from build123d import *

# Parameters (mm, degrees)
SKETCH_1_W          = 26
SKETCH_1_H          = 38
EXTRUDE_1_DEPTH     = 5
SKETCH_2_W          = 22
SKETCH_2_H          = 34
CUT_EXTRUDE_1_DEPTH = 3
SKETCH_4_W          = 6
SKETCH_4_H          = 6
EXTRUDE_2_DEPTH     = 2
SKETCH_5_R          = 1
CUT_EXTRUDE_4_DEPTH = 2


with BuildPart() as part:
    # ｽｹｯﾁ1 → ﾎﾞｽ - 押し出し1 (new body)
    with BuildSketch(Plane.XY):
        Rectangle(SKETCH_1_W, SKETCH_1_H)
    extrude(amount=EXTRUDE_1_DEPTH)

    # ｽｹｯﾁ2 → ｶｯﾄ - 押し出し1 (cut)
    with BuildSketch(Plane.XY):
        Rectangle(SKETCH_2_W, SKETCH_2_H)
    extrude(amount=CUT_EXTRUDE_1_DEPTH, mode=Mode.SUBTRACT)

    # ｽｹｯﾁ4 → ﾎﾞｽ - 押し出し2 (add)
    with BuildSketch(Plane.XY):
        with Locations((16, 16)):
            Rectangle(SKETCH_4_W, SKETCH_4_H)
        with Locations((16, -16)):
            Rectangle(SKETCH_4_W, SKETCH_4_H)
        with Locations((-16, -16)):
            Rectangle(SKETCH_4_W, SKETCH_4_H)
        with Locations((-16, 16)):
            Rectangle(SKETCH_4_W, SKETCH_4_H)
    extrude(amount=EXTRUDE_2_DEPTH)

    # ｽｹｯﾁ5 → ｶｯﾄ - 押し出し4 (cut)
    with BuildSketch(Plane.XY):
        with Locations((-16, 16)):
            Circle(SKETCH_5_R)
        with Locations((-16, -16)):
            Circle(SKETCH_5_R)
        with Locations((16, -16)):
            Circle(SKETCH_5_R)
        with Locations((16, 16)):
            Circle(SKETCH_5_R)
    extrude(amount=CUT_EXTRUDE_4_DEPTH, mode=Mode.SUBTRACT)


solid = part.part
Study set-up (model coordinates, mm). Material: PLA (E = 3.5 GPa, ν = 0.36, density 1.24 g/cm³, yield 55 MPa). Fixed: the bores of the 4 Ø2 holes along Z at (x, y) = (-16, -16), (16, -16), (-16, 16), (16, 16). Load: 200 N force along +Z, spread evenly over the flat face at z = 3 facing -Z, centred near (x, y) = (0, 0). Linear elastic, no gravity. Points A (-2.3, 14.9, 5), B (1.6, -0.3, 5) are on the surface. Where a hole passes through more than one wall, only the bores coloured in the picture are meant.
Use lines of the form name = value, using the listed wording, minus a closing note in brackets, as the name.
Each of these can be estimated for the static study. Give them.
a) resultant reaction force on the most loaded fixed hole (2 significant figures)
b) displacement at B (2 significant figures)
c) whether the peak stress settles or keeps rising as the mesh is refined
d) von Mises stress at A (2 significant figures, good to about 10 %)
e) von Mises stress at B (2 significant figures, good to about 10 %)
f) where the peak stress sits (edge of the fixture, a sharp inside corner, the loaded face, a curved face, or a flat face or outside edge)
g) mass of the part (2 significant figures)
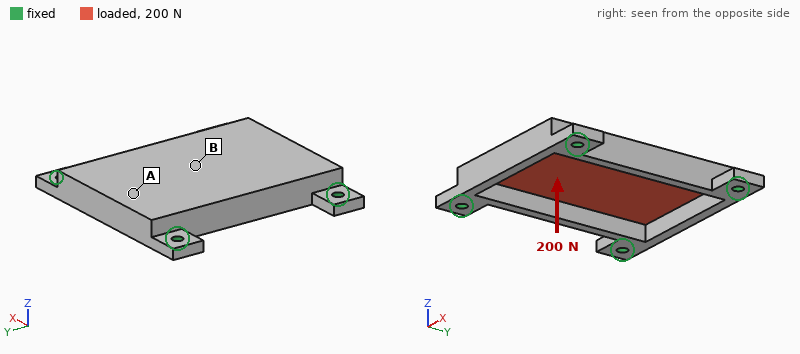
resultant reaction force on the most loaded fixed hole = 96 N
displacement at B = 0.30 mm
whether the peak stress settles or keeps rising as the mesh is refined = keeps rising
von Mises stress at A = 8.1 MPa
von Mises stress at B = 15 MPa
where the peak stress sits = edge of the fixture
mass of the part = 3.7 g
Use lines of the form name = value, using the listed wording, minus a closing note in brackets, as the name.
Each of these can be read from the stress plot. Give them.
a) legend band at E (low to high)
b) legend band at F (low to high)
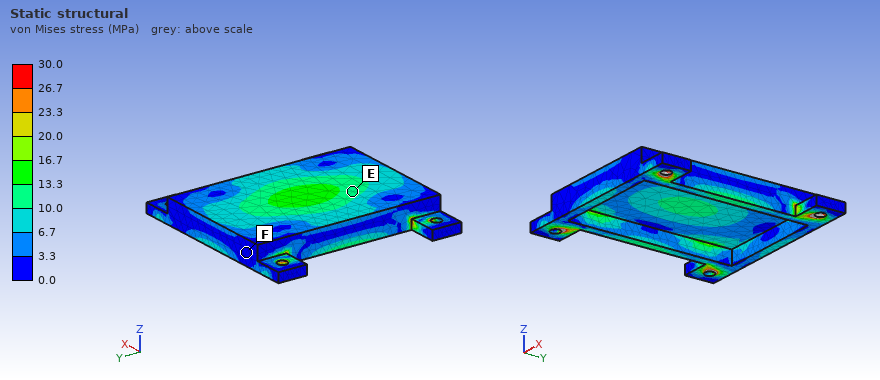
legend band at E = 10.0 to 13.3 MPa
legend band at F = 0.0 to 3.3 MPa
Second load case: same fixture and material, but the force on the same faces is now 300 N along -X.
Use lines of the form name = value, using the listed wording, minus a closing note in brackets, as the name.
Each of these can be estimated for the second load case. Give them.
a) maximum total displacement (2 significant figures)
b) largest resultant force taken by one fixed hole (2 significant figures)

maximum total displacement = 84 µm
largest resultant force taken by one fixed hole = 76 N
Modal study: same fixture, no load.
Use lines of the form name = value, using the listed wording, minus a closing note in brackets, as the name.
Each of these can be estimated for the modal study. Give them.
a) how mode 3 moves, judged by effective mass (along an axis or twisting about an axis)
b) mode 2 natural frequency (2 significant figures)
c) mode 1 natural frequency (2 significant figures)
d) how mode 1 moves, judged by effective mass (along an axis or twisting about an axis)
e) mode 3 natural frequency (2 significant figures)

how mode 3 moves, judged by effective mass = twisting about X
mode 2 natural frequency = 4800 Hz
mode 1 natural frequency = 3300 Hz
how mode 1 moves, judged by effective mass = along Z
mode 3 natural frequency = 5500 Hz
